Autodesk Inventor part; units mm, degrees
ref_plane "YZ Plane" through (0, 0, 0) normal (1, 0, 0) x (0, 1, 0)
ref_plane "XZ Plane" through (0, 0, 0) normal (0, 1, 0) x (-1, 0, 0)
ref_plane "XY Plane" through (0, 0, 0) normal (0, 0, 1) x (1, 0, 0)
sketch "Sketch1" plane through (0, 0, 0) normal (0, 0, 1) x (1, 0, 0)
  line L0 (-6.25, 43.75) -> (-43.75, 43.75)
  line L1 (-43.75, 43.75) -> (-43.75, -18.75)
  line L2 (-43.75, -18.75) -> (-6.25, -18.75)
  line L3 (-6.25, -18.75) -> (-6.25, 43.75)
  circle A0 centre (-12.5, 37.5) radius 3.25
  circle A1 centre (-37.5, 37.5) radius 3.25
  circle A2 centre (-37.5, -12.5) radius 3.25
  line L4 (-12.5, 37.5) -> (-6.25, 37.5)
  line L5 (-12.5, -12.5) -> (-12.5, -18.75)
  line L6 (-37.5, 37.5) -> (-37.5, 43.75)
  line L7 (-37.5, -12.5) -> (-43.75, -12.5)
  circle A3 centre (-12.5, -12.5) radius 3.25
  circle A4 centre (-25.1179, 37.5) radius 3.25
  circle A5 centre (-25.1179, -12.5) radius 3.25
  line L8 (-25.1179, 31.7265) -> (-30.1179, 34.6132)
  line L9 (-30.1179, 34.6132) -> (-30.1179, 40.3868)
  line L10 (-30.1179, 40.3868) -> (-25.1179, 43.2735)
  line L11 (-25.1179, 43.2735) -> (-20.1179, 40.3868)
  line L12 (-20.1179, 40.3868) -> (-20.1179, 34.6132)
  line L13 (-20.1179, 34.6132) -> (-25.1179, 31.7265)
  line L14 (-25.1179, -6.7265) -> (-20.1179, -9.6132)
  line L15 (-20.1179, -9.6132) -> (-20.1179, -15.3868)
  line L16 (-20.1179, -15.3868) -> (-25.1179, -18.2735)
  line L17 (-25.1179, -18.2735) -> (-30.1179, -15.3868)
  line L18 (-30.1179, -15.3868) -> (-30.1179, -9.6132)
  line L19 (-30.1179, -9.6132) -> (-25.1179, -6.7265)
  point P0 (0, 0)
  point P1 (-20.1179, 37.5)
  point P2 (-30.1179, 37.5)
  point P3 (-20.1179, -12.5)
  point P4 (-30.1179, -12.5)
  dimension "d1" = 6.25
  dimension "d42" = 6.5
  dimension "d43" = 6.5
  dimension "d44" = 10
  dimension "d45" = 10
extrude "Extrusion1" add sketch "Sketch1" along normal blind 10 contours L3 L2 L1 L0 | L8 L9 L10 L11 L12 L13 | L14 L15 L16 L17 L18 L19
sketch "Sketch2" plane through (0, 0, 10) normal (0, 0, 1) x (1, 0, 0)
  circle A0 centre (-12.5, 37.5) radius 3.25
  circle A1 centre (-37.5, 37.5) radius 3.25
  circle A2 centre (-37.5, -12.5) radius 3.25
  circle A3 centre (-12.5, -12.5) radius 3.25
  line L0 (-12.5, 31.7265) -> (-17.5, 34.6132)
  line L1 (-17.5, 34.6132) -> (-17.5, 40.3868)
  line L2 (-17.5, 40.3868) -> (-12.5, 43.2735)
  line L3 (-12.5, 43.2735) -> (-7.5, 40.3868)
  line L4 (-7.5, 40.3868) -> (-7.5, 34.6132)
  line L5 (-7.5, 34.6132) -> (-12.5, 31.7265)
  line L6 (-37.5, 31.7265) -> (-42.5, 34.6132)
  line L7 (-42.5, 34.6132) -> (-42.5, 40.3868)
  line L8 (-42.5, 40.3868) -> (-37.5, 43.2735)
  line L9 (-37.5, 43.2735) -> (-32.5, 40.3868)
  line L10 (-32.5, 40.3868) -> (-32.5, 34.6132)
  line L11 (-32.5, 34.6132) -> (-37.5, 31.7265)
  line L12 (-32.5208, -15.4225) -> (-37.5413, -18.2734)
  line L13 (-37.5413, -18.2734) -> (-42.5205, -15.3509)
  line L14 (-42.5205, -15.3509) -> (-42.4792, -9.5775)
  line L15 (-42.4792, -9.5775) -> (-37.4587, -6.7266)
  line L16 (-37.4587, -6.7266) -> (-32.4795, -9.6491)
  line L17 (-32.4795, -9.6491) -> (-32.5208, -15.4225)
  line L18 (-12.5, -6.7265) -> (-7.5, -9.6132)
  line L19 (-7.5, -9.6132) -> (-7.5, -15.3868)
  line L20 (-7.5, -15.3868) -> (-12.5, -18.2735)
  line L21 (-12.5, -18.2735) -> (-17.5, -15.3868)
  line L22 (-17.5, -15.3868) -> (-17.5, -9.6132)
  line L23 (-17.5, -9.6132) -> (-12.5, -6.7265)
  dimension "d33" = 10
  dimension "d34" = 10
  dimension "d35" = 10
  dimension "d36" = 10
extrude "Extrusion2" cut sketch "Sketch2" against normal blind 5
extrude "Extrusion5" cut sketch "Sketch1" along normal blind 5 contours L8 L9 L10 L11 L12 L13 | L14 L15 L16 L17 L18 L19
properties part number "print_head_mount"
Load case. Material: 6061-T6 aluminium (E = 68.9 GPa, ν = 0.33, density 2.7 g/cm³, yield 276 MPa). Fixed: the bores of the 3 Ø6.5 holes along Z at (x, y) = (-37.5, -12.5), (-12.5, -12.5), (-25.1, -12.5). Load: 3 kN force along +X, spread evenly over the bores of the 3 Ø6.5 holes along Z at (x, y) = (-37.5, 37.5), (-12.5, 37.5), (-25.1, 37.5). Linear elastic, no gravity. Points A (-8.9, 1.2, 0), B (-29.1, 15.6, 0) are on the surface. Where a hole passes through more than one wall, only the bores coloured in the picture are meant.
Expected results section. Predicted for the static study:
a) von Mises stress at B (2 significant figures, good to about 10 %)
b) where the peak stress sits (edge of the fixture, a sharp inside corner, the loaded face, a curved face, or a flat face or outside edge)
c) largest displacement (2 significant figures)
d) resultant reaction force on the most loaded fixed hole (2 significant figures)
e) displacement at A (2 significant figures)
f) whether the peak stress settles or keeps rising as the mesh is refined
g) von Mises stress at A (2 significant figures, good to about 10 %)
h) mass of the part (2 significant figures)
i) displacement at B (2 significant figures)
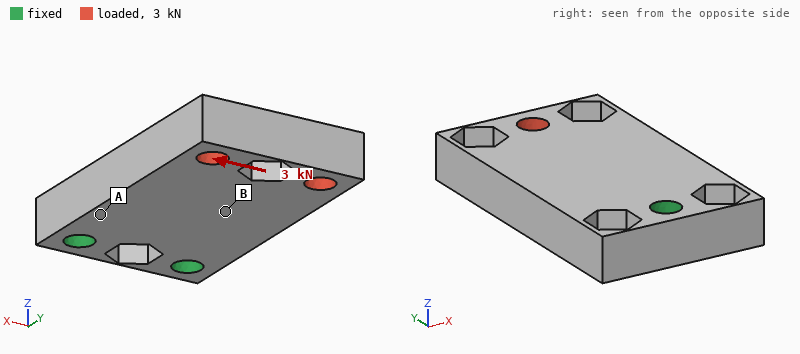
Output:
29 MPa
edge of the fixture
0.10 mm
5.2 kN
0.021 mm
keeps rising
55 MPa
54 g
0.037 mm
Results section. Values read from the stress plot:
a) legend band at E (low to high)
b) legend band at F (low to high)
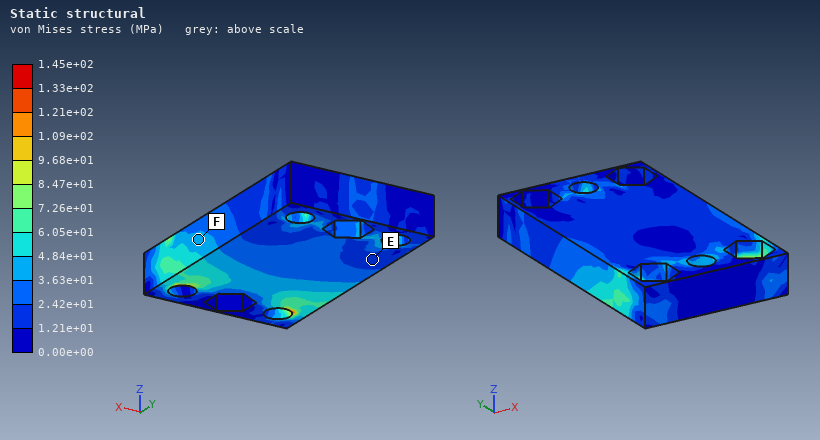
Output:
1.21e+01 to 2.42e+01 MPa
3.63e+01 to 4.84e+01 MPa
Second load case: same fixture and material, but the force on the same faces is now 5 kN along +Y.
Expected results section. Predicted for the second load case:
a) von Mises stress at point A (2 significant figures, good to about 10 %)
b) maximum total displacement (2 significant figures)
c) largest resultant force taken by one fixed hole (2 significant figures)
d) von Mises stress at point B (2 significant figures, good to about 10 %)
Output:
21 MPa
31 µm
1.8 kN
20 MPa
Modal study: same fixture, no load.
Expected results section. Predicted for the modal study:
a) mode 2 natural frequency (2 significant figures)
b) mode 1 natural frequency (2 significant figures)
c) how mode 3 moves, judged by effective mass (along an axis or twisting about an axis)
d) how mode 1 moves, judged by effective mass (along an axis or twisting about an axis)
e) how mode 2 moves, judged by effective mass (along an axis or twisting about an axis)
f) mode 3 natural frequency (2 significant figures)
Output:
7000 Hz
2600 Hz
along X
along Z
along X
8200 Hz
